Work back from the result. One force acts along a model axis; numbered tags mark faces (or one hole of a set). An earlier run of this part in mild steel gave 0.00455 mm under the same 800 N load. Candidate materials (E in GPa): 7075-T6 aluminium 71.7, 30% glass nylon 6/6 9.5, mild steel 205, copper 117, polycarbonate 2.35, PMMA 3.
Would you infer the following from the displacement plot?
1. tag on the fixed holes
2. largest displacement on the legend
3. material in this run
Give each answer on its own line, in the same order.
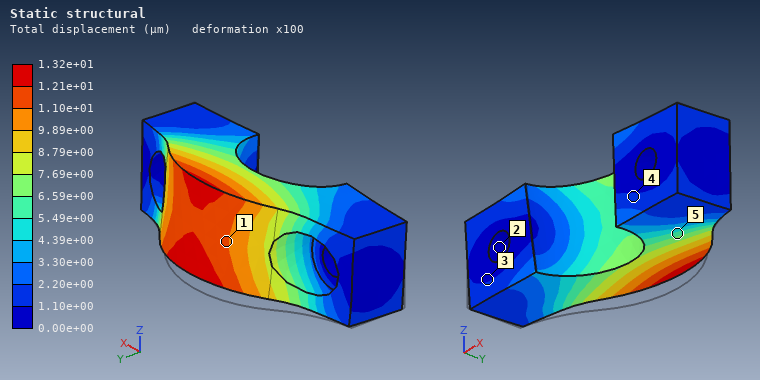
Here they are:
2
1.32e+01 µm
7075-T6 aluminium
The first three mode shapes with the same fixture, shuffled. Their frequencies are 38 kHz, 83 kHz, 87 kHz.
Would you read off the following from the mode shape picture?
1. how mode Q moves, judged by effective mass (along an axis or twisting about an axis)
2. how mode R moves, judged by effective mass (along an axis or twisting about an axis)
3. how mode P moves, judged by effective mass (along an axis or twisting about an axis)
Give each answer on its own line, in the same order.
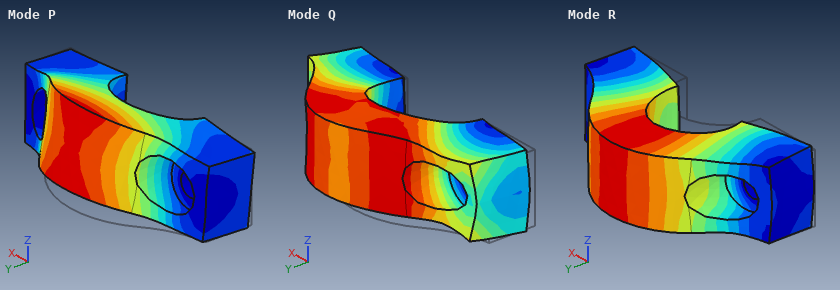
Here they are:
along X
along Y
along Z
